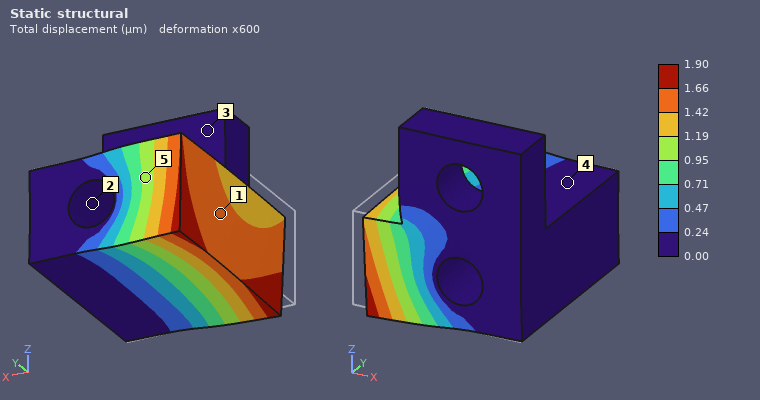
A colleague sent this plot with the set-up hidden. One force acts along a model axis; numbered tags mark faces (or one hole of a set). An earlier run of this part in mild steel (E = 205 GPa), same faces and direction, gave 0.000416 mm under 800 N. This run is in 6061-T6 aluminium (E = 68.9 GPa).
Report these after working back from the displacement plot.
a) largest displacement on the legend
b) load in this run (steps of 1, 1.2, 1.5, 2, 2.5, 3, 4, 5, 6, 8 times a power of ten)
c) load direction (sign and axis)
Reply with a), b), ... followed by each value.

a) 1.90 µm
b) 1.2 kN
c) +X
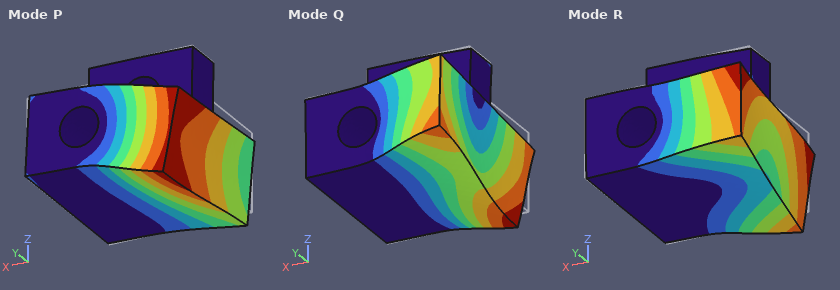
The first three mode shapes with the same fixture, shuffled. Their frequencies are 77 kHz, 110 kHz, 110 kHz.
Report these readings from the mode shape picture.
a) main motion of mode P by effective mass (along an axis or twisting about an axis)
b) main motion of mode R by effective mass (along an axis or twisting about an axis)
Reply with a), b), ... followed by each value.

a) along Z
b) along Y
